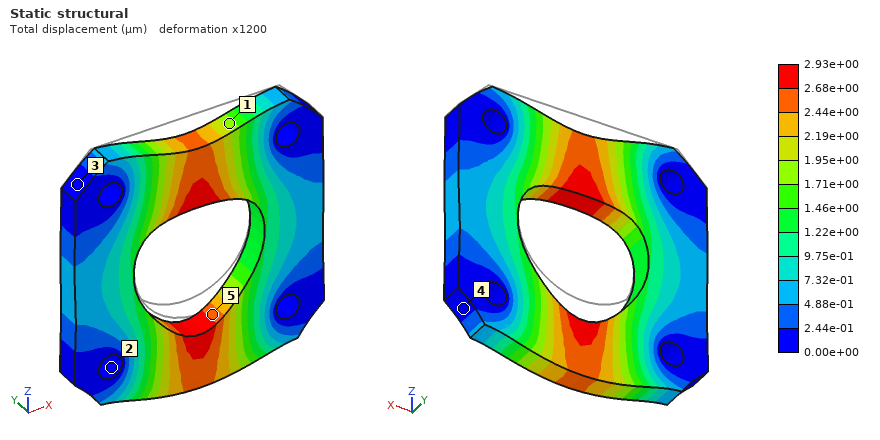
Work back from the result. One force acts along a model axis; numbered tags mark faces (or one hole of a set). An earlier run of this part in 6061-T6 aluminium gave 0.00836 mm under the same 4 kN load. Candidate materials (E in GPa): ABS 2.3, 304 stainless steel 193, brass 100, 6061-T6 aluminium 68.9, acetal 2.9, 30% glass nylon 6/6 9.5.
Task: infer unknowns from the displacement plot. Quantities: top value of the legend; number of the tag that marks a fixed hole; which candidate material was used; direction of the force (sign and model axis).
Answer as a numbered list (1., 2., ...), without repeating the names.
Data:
1. 2.93e+00 µm
2. 2
3. 304 stainless steel
4. -Z
